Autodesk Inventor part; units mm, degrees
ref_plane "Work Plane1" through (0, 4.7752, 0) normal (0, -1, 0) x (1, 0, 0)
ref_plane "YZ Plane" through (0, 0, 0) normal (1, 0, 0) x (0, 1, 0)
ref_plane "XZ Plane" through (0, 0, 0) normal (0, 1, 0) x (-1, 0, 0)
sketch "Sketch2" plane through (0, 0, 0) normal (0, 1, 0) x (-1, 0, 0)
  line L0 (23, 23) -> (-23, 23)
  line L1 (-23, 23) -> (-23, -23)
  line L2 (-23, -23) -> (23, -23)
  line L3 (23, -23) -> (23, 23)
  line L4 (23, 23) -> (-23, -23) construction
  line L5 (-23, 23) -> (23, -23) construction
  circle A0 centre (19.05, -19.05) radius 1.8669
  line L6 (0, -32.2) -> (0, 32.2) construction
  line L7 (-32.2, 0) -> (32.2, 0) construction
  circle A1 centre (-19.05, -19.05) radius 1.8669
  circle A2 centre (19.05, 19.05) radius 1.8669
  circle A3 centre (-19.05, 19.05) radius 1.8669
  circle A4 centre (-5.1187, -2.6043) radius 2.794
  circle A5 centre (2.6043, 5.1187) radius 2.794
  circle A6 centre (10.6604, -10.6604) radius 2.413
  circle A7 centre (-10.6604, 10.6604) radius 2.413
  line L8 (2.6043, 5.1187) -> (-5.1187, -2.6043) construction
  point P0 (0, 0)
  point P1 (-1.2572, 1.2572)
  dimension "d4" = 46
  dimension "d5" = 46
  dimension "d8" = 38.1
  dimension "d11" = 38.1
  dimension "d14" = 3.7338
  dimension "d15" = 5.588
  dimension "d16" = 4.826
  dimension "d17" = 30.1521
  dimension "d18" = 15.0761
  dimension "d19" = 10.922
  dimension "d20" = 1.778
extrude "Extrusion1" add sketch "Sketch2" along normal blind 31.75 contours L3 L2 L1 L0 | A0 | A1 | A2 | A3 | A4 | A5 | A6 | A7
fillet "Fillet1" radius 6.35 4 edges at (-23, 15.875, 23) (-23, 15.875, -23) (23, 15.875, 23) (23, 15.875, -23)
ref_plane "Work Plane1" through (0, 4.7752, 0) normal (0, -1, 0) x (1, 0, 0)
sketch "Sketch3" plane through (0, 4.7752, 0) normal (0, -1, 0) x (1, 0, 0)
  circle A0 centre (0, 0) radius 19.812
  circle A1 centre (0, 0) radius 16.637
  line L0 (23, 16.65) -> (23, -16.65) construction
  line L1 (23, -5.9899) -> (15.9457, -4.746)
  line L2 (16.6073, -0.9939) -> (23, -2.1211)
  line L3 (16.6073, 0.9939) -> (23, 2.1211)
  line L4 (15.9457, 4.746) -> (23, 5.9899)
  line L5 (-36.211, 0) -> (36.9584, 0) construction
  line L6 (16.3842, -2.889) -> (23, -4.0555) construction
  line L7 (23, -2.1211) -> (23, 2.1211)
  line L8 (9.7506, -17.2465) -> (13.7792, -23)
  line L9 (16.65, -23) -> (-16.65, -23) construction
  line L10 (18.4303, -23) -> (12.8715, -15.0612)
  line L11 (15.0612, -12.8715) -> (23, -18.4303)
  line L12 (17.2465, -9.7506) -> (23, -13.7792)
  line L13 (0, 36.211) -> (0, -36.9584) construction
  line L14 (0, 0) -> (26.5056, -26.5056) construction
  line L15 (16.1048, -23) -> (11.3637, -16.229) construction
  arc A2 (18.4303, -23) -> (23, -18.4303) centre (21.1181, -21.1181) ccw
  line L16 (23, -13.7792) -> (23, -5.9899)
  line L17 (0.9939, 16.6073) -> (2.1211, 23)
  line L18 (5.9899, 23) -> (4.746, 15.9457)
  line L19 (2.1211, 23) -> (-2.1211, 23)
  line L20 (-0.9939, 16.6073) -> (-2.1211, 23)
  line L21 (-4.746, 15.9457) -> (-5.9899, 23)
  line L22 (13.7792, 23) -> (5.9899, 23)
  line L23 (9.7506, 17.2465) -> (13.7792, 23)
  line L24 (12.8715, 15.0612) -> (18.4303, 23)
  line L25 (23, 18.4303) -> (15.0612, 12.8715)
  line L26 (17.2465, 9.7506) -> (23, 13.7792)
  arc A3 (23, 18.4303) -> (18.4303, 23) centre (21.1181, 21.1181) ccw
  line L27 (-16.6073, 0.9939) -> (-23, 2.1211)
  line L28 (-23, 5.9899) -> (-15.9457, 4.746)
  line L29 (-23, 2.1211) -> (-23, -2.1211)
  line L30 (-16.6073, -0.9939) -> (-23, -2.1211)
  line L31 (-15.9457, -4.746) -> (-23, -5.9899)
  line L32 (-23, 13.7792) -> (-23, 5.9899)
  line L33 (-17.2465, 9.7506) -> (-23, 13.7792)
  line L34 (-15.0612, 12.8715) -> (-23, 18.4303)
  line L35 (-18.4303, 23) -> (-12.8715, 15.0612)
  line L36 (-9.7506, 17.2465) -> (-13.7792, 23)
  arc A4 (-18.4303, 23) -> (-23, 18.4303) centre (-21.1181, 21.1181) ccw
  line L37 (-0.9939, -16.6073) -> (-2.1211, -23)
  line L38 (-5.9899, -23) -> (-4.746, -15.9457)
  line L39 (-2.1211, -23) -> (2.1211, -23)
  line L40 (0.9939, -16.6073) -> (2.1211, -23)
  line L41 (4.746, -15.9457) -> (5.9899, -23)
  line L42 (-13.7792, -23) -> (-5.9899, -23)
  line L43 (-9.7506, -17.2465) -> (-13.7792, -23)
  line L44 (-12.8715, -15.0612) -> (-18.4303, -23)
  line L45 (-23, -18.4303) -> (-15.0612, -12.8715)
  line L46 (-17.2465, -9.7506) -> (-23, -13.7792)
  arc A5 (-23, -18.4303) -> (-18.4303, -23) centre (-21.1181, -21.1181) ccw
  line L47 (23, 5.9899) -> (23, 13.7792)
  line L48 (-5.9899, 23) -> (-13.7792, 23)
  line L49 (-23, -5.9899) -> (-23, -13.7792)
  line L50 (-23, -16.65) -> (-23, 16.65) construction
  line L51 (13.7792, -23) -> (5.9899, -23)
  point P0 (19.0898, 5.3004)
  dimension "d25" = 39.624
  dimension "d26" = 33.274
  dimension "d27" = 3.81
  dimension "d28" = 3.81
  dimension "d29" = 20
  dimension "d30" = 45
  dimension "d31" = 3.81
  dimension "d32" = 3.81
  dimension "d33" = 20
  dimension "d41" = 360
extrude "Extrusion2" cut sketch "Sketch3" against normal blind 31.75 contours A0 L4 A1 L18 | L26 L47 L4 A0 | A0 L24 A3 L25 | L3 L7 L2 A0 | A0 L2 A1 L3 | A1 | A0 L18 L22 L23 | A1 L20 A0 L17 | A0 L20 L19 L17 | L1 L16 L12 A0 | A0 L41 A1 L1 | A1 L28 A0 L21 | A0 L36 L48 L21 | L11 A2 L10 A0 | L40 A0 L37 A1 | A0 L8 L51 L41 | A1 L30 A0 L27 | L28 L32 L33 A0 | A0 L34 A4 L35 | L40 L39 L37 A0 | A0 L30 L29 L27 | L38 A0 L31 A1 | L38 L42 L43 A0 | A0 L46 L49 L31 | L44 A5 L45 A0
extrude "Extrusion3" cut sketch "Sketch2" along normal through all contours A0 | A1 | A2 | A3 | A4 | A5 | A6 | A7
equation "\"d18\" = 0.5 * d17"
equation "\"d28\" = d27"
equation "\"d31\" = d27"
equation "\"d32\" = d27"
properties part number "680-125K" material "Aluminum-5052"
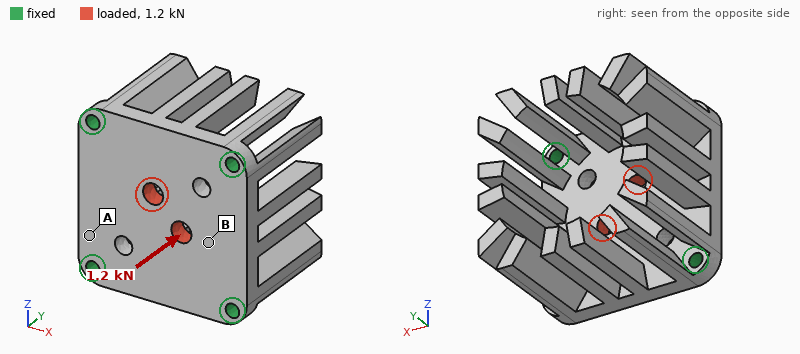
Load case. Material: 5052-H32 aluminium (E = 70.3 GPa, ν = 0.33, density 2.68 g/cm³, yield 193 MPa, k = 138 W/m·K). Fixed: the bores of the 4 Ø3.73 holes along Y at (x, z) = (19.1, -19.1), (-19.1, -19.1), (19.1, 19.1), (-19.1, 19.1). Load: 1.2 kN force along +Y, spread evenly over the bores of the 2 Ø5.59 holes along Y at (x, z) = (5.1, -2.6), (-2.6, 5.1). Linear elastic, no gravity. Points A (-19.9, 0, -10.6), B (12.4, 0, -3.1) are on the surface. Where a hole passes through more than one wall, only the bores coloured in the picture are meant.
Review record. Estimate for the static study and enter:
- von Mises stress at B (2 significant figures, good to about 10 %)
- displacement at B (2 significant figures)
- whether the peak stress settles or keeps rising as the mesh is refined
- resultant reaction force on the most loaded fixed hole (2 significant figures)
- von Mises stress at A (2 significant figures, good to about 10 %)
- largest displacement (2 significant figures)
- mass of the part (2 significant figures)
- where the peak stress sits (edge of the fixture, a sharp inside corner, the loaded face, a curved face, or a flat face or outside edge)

32 MPa
23 µm
keeps rising
330 N
14 MPa
48 µm
58 g
edge of the fixture
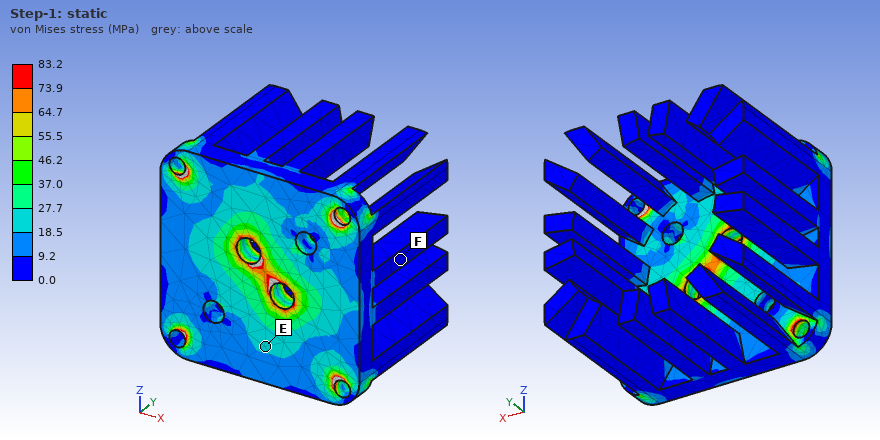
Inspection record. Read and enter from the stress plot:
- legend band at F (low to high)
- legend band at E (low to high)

0.0 to 9.2 MPa
18.5 to 27.7 MPa
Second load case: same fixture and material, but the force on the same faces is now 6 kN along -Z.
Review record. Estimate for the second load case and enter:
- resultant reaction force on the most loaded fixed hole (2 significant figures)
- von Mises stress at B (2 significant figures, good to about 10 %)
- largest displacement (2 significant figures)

1.8 kN
32 MPa
16 µm
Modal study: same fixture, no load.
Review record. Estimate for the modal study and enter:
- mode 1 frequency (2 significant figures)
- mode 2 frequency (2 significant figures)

3400 Hz
3500 Hz
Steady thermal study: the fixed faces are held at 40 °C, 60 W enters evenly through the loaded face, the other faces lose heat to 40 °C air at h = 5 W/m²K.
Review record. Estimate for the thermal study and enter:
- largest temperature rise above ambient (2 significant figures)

36 K
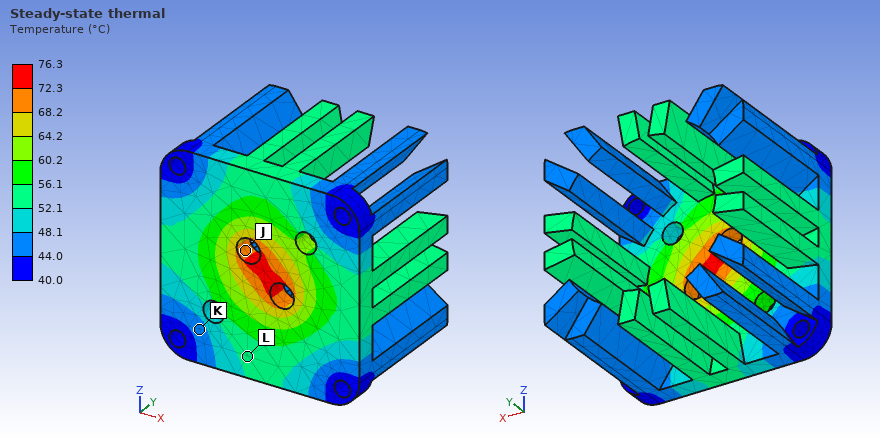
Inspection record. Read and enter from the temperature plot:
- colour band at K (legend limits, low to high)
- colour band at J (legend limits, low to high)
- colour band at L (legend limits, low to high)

44.0 to 48.1 °C
68.2 to 72.3 °C
52.1 to 56.1 °C
